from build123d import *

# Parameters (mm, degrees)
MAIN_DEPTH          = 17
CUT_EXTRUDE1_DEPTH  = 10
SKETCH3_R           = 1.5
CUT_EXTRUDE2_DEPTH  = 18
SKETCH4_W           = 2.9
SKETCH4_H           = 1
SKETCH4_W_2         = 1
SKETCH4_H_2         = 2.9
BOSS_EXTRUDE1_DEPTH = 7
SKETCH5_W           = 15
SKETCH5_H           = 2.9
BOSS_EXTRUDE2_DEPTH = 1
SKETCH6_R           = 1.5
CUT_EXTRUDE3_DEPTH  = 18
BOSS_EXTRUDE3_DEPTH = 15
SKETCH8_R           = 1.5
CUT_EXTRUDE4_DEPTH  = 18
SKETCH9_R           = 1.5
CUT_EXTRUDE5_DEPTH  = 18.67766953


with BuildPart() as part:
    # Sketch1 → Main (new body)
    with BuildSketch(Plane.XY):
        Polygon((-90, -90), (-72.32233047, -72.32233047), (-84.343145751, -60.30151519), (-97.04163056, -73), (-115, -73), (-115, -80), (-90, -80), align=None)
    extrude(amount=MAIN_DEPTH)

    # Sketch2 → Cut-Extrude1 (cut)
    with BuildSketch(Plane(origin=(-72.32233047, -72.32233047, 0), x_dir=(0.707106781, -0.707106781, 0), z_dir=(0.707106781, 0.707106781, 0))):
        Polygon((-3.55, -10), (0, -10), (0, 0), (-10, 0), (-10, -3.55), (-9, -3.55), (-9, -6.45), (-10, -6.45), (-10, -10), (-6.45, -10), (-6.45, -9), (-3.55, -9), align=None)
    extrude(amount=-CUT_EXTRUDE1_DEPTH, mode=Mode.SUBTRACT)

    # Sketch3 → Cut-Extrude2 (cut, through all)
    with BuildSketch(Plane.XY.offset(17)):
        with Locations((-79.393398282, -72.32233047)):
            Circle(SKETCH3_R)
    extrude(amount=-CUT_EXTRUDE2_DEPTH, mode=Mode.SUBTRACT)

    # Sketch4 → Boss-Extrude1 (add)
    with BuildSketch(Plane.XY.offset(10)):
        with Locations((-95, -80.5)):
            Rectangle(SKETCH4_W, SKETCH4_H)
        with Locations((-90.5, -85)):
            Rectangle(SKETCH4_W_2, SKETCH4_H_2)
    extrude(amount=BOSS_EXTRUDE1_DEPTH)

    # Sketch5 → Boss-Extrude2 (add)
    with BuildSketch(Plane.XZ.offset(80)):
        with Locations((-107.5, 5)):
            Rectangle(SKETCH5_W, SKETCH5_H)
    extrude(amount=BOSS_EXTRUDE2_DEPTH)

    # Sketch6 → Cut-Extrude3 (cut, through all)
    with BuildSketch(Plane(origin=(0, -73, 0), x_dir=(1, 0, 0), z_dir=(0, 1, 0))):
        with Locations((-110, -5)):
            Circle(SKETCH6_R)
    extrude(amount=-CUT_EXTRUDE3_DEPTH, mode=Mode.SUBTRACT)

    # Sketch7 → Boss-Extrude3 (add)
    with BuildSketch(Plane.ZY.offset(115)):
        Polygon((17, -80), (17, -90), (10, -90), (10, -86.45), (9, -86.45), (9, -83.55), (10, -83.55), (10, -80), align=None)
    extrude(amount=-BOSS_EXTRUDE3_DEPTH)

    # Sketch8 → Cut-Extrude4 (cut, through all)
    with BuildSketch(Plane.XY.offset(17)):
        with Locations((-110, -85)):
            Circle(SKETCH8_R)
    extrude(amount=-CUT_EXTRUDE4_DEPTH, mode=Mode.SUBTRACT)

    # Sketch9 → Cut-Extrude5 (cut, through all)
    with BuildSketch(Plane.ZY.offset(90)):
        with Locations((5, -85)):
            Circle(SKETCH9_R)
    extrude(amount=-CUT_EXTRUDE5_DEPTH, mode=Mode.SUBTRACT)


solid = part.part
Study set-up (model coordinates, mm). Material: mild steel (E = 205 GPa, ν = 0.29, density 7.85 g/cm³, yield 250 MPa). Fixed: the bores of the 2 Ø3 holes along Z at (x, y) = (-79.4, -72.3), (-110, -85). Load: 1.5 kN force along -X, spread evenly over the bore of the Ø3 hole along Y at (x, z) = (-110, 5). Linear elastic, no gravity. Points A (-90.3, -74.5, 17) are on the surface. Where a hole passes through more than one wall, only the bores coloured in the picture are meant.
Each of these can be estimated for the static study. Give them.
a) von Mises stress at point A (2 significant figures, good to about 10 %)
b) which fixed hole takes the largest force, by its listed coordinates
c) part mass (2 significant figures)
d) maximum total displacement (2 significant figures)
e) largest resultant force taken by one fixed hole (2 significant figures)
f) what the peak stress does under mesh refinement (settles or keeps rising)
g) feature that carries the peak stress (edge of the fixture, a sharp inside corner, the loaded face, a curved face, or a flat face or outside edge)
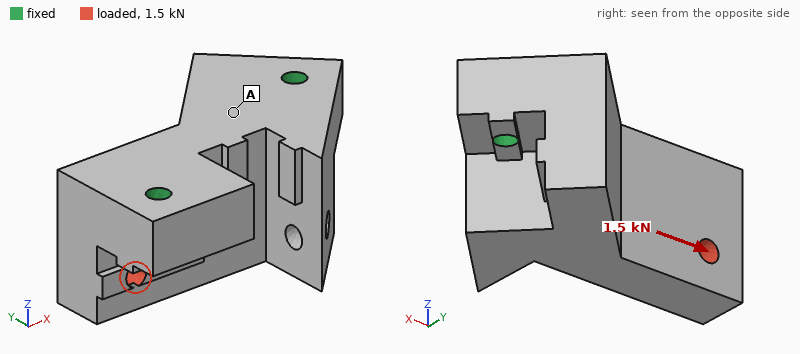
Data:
8.7 MPa
(-79.4, -72.3)
64 g
5.3 µm
1.1 kN
keeps rising
a sharp inside corner
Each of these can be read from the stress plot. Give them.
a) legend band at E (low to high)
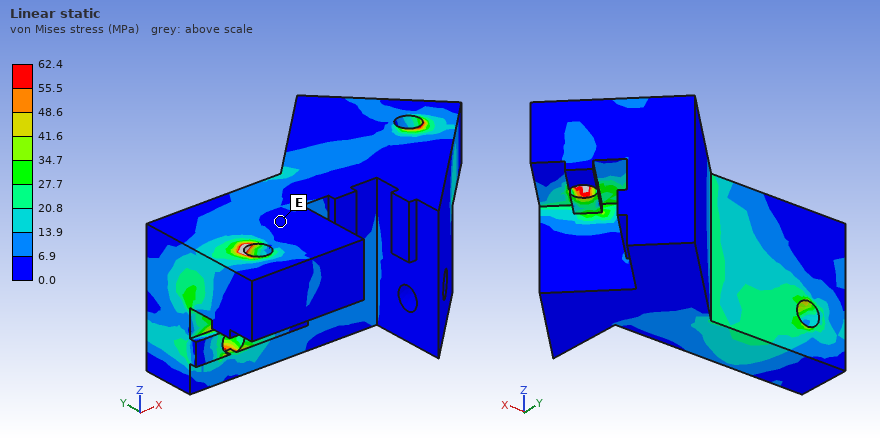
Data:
0.0 to 6.9 MPa
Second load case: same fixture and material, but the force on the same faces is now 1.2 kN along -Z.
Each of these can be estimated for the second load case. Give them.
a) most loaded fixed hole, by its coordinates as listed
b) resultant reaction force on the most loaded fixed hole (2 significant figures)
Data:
(-110, -85)
1.1 kN
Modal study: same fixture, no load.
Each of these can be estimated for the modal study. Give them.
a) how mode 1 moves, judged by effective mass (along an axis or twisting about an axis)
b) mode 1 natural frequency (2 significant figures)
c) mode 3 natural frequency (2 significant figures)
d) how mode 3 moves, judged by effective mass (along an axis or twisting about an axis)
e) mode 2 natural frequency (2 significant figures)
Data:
along Y
12 kHz
21 kHz
along Z
19 kHz
